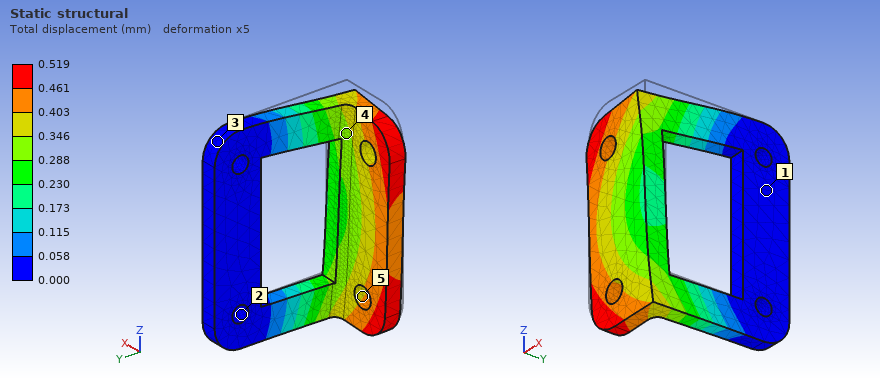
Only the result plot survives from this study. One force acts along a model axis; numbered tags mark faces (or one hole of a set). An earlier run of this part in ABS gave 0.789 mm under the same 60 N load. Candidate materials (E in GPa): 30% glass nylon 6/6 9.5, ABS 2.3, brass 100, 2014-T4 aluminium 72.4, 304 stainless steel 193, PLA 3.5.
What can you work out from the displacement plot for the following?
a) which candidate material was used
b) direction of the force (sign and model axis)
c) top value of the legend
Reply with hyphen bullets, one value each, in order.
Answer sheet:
- PLA
- -Z
- 0.519 mm
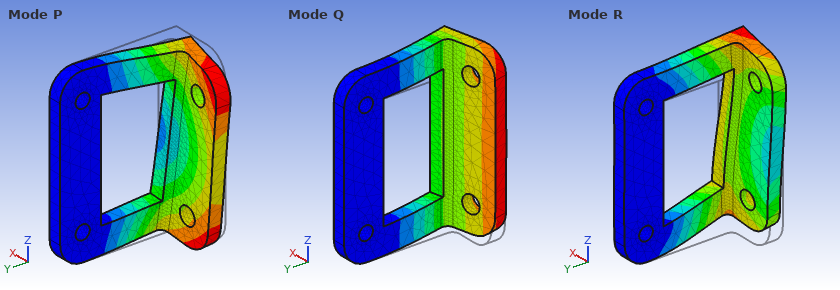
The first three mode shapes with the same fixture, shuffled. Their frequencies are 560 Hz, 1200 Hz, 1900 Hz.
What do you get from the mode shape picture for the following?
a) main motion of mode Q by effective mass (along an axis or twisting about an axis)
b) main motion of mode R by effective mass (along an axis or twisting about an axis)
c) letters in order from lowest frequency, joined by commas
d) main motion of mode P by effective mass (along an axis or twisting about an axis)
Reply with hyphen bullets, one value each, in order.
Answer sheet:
- along X
- along Z
- Q, P, R
- along Z
